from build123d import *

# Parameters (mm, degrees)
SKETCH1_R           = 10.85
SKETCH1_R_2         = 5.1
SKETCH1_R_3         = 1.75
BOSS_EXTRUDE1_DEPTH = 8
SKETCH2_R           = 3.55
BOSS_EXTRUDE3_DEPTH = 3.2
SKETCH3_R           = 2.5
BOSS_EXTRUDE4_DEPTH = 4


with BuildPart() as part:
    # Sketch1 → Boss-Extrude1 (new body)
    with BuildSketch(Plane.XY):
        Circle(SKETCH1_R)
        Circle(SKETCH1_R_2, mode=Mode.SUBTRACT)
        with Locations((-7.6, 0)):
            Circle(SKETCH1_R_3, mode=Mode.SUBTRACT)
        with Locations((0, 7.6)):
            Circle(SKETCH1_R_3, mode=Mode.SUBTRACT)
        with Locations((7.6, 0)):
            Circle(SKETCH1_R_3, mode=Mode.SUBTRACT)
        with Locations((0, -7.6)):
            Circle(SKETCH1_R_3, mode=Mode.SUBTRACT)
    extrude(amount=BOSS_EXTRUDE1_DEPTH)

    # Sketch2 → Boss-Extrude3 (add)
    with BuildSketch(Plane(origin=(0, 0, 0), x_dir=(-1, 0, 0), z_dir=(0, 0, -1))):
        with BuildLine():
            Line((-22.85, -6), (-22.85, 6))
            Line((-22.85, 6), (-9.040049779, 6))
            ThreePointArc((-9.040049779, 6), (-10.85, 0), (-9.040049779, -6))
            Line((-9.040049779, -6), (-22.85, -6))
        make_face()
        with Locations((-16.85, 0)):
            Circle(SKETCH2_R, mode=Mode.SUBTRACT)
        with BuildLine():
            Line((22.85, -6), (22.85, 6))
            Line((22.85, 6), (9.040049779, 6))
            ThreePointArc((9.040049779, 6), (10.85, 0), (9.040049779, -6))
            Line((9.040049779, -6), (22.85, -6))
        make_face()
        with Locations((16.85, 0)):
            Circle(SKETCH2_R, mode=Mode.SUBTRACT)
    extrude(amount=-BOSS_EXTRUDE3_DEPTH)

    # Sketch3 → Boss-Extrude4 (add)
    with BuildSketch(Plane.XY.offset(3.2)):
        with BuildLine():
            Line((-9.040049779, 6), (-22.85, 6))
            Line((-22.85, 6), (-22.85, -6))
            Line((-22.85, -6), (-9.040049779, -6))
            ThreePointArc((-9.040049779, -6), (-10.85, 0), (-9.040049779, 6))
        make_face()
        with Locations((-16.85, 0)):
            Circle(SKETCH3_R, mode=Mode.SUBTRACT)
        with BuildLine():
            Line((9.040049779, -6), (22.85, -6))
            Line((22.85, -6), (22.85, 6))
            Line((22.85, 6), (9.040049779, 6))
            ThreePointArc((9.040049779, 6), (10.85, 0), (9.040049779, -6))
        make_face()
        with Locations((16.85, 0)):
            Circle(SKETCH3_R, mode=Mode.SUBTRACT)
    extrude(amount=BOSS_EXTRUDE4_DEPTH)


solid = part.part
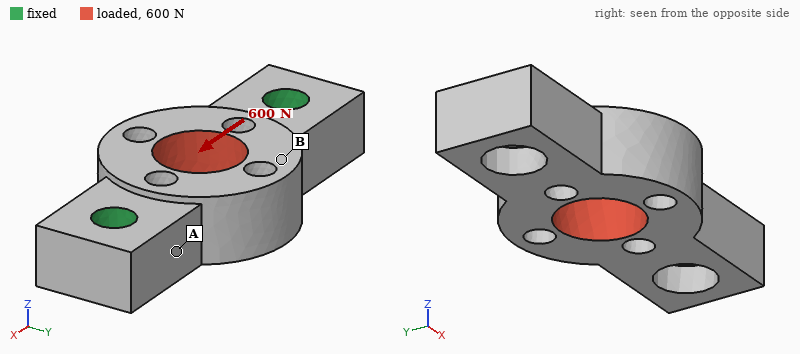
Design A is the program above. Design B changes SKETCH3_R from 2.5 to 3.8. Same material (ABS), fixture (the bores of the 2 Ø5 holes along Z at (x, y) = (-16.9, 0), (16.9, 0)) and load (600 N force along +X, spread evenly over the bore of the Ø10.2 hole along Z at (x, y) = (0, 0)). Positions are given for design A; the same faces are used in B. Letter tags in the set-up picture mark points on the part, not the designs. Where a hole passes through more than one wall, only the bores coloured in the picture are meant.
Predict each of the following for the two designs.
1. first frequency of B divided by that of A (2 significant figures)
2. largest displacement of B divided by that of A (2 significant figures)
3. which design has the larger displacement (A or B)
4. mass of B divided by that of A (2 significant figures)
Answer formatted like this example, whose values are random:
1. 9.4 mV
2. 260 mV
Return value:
1. 1.2
2. 0.83
3. A
4. 0.95
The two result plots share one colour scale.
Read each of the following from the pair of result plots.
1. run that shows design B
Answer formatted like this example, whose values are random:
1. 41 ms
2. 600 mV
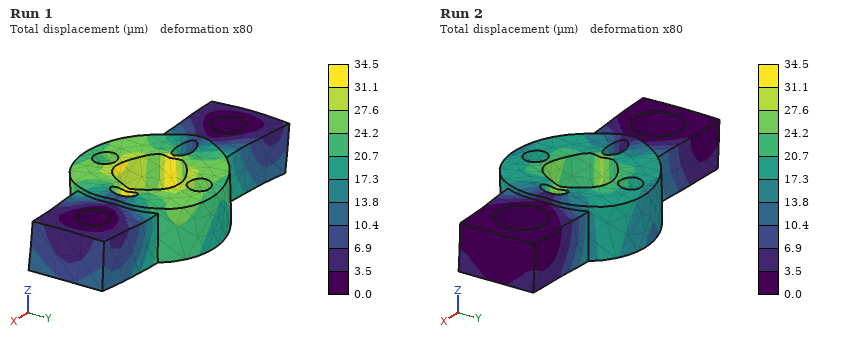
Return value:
1. Run 2
